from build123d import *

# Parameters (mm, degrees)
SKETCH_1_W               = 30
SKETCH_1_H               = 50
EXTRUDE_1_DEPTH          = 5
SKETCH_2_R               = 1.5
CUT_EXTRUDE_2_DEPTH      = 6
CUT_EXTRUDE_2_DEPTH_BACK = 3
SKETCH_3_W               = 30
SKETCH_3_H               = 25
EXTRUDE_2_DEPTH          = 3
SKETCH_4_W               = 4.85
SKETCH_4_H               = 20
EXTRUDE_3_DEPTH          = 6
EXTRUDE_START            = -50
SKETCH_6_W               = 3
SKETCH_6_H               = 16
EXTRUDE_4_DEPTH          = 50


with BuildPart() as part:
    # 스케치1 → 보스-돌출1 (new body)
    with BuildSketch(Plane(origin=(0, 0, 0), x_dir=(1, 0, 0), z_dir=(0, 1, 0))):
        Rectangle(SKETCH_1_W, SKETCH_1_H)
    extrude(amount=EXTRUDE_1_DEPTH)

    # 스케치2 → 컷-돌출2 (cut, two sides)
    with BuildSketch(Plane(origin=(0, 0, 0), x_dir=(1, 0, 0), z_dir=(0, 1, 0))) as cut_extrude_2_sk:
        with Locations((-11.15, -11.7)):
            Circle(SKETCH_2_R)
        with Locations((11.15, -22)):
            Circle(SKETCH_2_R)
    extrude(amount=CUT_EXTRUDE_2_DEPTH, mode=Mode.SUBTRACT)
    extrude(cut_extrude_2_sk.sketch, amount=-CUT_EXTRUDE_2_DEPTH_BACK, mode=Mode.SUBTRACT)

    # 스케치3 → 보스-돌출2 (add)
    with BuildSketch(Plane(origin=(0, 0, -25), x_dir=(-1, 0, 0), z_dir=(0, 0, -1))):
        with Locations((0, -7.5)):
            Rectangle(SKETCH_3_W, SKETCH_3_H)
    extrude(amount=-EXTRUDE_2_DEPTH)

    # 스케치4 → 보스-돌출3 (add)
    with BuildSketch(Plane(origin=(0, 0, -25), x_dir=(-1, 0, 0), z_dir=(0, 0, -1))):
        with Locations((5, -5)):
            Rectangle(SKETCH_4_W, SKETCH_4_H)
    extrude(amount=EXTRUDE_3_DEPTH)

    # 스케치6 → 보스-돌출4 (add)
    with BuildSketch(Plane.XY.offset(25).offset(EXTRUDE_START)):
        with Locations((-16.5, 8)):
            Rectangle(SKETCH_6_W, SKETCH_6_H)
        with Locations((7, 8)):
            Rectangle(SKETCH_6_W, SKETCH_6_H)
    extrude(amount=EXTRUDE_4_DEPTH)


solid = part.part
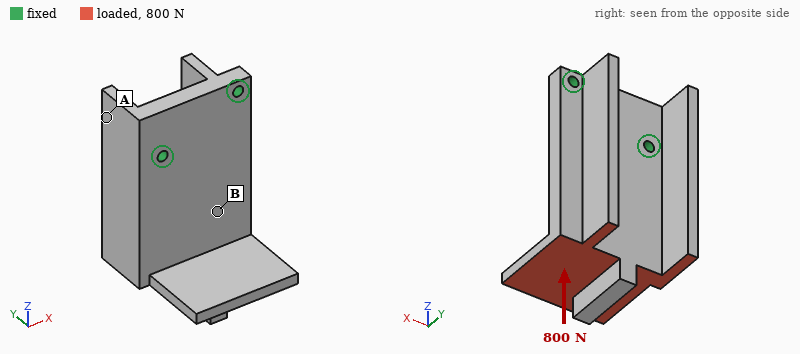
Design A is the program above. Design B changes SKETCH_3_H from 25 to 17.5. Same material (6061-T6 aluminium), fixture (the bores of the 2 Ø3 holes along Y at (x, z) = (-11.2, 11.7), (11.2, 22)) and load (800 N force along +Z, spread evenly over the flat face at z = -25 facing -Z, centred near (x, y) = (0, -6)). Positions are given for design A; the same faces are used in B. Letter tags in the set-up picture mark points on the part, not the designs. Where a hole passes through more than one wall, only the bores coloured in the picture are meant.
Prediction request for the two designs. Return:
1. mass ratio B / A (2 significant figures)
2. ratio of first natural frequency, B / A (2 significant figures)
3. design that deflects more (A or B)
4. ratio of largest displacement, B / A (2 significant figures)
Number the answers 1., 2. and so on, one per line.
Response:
1. 0.98
2. 1.0
3. A
4. 0.66
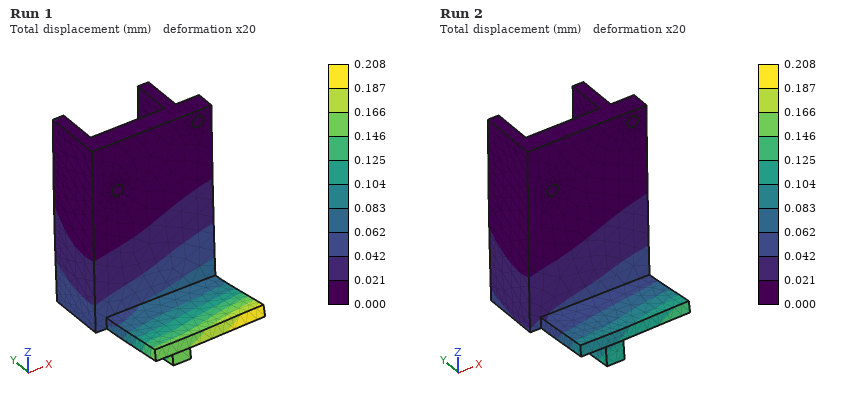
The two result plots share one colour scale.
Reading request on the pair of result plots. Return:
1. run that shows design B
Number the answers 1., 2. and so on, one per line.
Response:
1. Run 2
